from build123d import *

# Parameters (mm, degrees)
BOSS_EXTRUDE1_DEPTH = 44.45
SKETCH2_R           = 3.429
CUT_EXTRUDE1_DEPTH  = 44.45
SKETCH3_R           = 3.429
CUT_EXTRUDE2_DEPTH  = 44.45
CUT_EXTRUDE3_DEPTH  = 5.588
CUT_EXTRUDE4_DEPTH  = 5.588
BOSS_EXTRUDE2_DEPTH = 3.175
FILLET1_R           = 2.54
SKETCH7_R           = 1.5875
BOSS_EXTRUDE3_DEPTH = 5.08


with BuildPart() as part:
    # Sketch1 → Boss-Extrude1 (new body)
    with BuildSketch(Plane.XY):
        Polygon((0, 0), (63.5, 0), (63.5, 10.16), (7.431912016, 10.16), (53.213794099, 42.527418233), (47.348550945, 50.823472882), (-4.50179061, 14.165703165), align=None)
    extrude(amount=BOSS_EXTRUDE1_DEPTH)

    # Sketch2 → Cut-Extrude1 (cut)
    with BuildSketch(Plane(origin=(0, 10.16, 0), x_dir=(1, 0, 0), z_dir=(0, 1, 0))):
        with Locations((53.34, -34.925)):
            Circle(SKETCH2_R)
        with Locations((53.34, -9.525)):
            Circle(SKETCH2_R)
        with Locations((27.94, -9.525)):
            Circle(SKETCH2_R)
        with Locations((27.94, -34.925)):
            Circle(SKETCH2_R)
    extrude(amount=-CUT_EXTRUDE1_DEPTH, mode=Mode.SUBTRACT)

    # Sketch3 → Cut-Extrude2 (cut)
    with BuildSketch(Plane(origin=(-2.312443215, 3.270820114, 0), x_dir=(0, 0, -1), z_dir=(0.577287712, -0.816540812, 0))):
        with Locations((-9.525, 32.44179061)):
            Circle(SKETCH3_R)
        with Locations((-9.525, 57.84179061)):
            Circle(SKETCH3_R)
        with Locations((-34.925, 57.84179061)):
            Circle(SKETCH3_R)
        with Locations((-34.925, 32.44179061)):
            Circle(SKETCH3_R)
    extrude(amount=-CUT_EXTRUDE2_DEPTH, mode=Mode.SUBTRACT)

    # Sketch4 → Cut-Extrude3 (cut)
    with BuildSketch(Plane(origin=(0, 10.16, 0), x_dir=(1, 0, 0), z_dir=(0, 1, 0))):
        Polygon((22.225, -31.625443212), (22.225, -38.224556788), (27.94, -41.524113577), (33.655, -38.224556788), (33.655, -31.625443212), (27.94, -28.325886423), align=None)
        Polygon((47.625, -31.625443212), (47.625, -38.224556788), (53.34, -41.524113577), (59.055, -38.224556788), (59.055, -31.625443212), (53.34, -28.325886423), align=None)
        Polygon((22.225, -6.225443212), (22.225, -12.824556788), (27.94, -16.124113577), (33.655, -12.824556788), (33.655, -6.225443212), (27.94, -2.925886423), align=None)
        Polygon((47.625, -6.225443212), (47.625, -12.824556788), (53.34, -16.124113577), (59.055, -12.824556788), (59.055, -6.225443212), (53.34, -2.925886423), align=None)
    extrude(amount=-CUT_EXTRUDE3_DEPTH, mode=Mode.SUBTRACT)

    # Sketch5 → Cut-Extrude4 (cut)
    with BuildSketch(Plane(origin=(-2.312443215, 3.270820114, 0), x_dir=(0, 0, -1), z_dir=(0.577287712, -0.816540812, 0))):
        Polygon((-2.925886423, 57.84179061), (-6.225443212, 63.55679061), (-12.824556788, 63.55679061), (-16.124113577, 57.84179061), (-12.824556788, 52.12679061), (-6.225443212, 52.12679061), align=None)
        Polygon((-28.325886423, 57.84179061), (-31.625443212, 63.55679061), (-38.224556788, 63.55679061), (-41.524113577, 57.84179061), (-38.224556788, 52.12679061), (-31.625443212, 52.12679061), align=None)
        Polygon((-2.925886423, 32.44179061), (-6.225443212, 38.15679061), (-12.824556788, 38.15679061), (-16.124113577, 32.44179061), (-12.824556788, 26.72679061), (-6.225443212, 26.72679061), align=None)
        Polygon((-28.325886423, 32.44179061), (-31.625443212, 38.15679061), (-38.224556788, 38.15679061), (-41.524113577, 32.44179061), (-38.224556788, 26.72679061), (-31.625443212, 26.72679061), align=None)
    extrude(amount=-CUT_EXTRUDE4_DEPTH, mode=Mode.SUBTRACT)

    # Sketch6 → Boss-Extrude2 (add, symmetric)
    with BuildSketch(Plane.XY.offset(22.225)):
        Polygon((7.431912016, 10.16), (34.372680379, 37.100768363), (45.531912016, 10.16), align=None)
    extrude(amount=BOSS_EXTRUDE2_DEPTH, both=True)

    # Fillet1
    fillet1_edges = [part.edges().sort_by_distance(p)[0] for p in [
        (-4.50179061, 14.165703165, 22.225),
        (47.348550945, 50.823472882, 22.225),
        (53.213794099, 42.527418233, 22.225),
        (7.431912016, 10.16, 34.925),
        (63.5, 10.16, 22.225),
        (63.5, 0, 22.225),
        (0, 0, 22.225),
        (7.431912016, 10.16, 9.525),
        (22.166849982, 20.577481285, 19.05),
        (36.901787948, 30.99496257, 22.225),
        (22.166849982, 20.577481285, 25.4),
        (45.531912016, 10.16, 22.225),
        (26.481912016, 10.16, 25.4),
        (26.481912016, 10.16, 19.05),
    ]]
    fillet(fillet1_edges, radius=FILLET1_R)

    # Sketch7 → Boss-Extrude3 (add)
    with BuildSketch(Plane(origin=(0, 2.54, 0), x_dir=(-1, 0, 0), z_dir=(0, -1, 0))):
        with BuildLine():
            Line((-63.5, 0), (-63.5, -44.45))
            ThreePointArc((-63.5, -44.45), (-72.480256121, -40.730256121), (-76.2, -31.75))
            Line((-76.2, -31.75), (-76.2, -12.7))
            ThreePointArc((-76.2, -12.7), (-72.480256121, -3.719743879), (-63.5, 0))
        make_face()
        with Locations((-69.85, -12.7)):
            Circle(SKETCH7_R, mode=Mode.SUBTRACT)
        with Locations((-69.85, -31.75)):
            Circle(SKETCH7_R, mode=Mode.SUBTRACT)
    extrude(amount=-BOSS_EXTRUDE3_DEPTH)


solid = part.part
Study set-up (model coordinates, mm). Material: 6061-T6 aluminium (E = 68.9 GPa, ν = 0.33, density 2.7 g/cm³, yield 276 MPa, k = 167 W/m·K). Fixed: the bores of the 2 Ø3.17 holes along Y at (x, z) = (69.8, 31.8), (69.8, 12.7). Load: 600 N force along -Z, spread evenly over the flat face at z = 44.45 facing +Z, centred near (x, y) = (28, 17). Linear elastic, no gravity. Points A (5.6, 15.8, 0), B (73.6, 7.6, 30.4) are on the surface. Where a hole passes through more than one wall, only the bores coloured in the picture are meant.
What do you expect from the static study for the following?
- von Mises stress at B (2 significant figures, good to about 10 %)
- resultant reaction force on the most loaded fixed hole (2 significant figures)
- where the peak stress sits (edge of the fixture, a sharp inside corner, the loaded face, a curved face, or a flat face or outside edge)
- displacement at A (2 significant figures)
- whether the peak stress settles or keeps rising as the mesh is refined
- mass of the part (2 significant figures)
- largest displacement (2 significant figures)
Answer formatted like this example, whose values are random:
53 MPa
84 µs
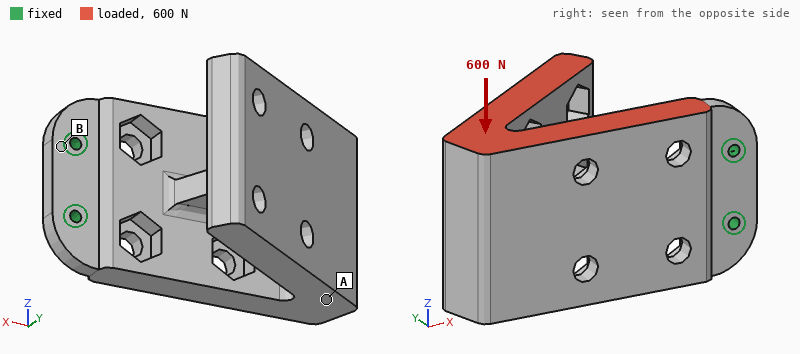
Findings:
11 MPa
1.3 kN
edge of the fixture
58 µm
keeps rising
150 g
90 µm
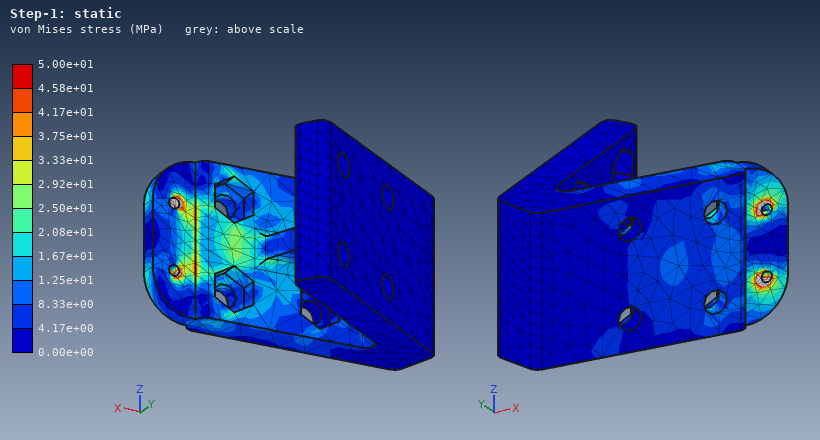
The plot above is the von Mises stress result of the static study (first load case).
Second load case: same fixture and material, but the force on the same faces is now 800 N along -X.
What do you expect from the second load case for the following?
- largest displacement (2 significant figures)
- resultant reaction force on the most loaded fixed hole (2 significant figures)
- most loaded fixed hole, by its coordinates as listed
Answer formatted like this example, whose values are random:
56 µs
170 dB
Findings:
0.26 mm
1.2 kN
(69.8, 31.8)
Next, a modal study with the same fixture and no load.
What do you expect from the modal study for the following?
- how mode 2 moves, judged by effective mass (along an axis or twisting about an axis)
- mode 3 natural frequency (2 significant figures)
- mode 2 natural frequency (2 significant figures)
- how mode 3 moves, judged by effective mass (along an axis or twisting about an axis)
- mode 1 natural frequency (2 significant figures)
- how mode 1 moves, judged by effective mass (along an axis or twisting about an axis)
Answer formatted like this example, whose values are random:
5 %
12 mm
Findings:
along Z
2400 Hz
1300 Hz
along Z
470 Hz
along Y
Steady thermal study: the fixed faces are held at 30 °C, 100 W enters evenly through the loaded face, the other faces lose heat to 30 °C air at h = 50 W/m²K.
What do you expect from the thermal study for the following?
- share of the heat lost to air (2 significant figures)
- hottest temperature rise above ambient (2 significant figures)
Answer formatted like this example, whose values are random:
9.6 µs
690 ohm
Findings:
37 %
69 K
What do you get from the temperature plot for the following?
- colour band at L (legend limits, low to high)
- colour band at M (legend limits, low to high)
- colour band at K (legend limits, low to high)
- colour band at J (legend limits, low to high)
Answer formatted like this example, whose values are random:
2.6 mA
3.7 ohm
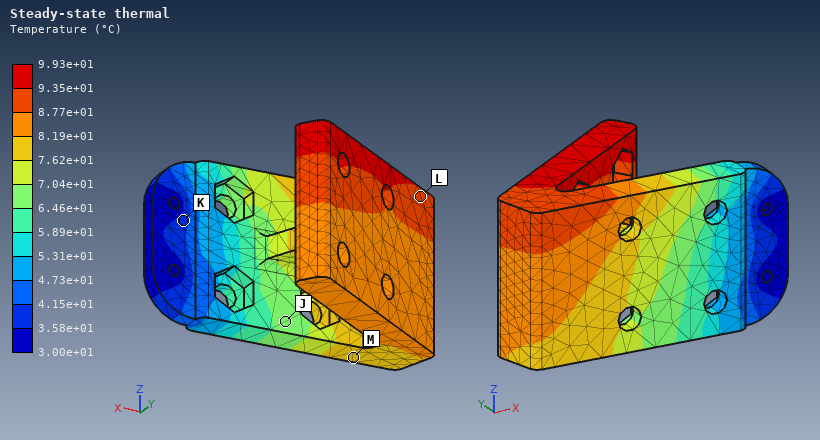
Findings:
8.77e+01 to 9.35e+01 °C
7.62e+01 to 8.19e+01 °C
3.58e+01 to 4.15e+01 °C
6.46e+01 to 7.04e+01 °C
